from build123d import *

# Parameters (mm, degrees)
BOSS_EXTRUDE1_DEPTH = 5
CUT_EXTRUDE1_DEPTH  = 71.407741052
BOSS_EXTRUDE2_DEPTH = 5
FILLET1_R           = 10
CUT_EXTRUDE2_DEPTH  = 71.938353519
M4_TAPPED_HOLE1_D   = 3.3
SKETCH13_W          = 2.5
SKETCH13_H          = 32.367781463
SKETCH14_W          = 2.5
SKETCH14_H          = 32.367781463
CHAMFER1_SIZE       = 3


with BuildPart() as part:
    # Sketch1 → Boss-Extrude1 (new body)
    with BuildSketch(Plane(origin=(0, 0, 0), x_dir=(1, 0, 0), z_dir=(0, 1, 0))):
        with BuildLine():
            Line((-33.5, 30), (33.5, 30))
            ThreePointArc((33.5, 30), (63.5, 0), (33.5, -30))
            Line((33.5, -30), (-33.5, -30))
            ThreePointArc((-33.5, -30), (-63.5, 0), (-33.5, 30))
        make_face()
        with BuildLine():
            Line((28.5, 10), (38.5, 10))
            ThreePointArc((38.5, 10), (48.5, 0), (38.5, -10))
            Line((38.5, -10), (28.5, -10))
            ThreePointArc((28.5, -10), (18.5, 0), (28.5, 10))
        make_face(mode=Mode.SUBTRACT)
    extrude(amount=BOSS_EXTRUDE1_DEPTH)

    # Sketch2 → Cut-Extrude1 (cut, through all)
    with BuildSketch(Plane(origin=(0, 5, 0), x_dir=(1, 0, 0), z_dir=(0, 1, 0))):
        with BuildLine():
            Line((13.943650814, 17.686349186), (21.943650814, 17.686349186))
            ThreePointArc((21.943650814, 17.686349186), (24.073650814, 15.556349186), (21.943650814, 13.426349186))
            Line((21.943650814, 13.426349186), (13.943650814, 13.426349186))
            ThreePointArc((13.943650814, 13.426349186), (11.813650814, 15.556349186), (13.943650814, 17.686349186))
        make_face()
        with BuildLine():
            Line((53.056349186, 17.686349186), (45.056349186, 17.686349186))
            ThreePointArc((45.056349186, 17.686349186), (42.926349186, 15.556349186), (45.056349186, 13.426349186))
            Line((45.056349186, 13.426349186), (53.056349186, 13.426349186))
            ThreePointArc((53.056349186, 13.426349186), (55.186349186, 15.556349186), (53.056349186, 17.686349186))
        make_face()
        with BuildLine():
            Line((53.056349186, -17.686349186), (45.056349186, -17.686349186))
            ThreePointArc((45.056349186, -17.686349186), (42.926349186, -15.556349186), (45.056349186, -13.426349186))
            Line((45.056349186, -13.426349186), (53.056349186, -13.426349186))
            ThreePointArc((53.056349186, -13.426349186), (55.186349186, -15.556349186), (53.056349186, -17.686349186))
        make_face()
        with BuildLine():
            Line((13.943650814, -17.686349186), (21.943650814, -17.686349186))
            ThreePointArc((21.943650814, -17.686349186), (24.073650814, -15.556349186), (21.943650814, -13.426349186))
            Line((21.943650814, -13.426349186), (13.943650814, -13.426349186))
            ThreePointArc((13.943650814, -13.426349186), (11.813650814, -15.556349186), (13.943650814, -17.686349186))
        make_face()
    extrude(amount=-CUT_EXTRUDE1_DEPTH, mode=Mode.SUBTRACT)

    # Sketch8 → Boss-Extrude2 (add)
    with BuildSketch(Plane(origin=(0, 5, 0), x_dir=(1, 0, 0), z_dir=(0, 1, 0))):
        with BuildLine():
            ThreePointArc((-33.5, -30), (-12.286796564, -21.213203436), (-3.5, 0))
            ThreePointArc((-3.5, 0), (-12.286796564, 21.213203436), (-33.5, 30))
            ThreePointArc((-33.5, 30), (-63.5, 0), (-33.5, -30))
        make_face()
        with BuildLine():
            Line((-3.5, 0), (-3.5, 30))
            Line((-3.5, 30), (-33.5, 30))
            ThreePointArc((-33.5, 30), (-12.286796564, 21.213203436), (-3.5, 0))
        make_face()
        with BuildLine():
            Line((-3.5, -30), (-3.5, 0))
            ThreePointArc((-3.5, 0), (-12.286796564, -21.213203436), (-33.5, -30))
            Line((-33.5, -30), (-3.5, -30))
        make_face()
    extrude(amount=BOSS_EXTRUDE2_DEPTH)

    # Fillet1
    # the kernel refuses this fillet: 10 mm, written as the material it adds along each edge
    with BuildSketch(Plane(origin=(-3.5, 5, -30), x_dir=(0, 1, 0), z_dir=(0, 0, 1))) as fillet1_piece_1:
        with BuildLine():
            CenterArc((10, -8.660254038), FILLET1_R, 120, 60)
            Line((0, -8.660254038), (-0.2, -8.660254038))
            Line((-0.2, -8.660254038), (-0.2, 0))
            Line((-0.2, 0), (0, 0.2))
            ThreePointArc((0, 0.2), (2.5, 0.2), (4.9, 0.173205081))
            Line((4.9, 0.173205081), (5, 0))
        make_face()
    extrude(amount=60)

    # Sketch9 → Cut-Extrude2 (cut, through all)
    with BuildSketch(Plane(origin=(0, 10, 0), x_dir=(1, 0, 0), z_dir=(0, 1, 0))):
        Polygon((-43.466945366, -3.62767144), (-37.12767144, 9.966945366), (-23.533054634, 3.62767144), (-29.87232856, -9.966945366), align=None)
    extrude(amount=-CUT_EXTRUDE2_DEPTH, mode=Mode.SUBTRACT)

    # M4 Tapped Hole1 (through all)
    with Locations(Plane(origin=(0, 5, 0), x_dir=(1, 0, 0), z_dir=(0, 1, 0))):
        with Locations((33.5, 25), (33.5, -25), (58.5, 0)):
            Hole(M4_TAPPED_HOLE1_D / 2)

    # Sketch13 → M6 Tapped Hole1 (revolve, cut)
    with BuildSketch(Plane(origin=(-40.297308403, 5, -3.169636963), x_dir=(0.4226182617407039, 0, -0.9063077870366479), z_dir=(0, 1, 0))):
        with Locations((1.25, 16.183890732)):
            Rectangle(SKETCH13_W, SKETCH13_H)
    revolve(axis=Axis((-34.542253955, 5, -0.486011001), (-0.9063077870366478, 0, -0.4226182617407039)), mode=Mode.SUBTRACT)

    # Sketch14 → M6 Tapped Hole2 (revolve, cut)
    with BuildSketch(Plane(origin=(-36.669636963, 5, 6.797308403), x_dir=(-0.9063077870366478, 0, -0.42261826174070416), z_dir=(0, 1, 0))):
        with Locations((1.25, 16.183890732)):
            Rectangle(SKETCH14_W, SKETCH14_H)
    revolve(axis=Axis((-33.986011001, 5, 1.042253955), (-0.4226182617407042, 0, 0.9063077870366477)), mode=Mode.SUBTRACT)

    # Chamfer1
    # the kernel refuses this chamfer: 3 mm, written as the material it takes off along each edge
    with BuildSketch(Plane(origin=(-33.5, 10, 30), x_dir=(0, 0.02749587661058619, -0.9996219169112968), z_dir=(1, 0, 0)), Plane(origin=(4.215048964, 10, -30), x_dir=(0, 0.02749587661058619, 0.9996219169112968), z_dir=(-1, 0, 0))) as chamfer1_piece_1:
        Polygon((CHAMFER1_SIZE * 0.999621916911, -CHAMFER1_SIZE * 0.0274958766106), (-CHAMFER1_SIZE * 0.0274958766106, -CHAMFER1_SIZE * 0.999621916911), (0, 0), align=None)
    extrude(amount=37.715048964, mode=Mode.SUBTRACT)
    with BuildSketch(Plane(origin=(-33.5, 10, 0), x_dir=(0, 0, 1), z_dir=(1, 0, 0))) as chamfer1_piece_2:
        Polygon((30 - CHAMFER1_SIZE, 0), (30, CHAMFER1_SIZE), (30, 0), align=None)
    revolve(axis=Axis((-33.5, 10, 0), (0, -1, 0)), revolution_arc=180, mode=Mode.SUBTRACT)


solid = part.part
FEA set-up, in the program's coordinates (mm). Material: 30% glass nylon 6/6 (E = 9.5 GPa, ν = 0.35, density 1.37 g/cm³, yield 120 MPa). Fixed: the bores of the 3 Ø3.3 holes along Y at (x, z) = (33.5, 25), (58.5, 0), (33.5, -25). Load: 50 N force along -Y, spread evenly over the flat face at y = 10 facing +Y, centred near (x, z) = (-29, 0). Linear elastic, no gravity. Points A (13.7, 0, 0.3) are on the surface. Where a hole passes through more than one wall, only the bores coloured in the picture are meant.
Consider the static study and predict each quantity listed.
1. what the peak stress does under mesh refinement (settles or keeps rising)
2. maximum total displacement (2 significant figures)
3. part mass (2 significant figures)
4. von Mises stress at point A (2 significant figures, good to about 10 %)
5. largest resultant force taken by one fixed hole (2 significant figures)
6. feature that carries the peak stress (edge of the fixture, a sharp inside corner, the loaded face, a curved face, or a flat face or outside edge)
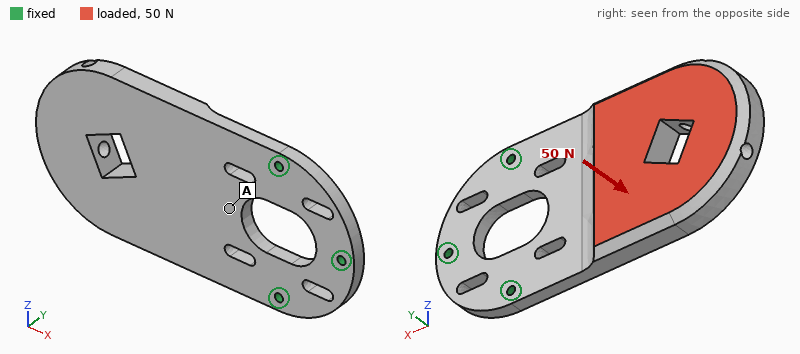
keeps rising
1.6 mm
60 g
4.3 MPa
42 N
edge of the fixture
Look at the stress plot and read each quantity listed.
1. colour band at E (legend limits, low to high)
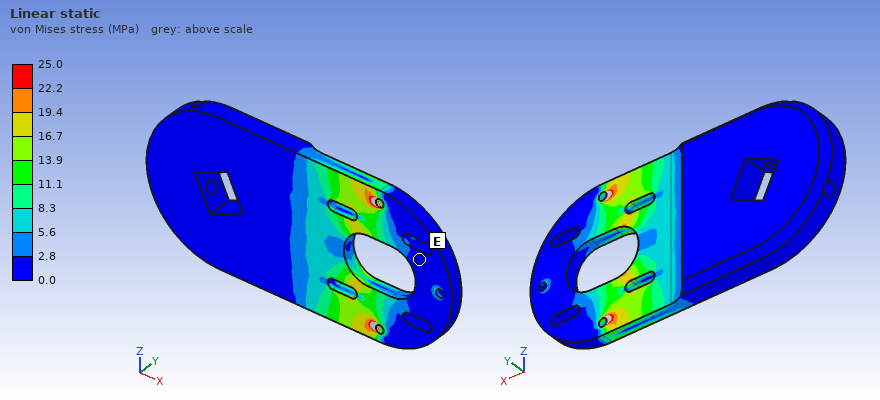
0.0 to 2.8 MPa
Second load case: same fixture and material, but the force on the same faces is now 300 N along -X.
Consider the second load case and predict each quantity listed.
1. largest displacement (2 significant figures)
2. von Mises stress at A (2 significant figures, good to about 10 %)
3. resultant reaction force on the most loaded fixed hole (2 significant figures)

1.5 mm
4.6 MPa
140 N
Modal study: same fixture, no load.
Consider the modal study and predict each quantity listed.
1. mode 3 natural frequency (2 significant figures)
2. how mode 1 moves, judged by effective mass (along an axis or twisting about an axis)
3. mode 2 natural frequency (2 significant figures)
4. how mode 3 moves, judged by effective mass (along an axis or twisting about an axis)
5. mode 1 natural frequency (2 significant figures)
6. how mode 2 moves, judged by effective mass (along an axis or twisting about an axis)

1700 Hz
along Y
950 Hz
along Z
170 Hz
twisting about X
